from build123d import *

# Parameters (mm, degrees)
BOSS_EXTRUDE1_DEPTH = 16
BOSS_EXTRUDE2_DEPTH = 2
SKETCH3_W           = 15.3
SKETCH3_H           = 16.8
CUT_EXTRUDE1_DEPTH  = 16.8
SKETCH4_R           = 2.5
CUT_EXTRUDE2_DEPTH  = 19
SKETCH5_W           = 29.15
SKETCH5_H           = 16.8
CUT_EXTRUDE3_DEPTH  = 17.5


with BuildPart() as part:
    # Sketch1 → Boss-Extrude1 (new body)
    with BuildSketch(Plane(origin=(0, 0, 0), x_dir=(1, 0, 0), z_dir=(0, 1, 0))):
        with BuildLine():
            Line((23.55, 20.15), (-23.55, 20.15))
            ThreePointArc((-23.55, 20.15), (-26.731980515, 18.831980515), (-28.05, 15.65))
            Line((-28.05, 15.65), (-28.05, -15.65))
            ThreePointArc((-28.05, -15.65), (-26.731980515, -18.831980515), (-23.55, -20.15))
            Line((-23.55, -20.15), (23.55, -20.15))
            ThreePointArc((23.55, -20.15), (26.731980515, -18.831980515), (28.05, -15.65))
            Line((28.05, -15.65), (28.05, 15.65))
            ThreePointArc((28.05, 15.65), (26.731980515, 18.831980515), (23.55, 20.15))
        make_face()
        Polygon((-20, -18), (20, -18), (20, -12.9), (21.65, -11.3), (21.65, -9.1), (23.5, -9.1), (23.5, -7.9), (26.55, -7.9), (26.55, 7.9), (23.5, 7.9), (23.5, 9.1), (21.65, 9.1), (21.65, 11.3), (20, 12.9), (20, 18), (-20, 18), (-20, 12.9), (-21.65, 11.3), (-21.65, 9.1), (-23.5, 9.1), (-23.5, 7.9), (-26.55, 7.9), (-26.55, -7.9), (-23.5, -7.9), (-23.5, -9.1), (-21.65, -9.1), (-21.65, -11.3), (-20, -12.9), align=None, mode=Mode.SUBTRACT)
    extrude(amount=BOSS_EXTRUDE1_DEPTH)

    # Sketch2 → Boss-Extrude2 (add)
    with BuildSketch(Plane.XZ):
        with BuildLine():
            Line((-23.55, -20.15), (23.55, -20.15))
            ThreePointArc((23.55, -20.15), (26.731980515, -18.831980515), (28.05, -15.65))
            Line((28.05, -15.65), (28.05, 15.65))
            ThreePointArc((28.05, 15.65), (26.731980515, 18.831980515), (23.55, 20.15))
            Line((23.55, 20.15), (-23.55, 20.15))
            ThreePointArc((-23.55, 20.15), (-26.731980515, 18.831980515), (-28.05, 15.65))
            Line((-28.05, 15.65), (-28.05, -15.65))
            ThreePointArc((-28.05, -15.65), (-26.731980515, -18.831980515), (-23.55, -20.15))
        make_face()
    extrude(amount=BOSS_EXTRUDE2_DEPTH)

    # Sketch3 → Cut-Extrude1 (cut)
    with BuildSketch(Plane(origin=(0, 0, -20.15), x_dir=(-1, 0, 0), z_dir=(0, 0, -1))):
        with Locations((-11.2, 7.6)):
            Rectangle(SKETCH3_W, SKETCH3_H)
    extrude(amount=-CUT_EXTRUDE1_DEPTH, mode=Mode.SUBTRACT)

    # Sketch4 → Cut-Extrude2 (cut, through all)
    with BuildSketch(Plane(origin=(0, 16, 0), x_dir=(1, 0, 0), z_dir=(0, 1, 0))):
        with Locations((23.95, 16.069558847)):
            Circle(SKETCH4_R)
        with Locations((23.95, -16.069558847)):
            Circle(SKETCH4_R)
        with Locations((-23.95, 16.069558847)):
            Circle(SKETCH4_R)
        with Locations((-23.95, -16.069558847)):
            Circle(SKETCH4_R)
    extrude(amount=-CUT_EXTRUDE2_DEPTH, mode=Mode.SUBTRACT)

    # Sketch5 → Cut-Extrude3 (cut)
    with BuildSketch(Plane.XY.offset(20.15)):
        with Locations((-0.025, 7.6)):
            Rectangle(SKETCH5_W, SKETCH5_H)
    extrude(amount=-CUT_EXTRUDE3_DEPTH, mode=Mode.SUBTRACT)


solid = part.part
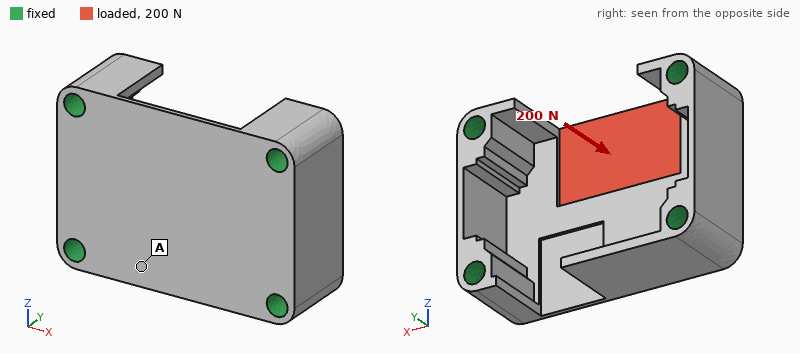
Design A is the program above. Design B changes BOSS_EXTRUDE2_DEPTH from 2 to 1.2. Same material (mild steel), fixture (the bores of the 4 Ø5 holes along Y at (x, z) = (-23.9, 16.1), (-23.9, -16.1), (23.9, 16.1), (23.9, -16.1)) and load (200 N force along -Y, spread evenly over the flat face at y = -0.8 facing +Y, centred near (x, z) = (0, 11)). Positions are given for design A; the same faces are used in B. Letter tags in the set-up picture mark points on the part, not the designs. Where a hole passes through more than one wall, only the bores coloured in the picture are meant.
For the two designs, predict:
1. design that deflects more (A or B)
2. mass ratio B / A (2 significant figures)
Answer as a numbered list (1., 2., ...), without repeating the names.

1. B
2. 0.82
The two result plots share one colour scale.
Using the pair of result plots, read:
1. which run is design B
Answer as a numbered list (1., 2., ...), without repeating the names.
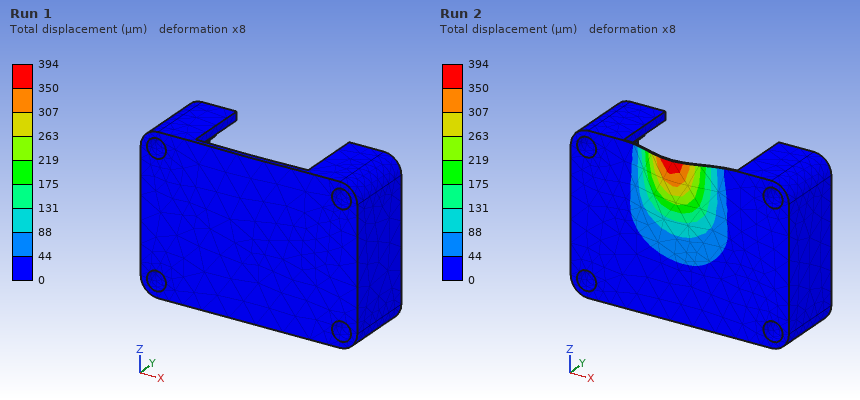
1. Run 2
